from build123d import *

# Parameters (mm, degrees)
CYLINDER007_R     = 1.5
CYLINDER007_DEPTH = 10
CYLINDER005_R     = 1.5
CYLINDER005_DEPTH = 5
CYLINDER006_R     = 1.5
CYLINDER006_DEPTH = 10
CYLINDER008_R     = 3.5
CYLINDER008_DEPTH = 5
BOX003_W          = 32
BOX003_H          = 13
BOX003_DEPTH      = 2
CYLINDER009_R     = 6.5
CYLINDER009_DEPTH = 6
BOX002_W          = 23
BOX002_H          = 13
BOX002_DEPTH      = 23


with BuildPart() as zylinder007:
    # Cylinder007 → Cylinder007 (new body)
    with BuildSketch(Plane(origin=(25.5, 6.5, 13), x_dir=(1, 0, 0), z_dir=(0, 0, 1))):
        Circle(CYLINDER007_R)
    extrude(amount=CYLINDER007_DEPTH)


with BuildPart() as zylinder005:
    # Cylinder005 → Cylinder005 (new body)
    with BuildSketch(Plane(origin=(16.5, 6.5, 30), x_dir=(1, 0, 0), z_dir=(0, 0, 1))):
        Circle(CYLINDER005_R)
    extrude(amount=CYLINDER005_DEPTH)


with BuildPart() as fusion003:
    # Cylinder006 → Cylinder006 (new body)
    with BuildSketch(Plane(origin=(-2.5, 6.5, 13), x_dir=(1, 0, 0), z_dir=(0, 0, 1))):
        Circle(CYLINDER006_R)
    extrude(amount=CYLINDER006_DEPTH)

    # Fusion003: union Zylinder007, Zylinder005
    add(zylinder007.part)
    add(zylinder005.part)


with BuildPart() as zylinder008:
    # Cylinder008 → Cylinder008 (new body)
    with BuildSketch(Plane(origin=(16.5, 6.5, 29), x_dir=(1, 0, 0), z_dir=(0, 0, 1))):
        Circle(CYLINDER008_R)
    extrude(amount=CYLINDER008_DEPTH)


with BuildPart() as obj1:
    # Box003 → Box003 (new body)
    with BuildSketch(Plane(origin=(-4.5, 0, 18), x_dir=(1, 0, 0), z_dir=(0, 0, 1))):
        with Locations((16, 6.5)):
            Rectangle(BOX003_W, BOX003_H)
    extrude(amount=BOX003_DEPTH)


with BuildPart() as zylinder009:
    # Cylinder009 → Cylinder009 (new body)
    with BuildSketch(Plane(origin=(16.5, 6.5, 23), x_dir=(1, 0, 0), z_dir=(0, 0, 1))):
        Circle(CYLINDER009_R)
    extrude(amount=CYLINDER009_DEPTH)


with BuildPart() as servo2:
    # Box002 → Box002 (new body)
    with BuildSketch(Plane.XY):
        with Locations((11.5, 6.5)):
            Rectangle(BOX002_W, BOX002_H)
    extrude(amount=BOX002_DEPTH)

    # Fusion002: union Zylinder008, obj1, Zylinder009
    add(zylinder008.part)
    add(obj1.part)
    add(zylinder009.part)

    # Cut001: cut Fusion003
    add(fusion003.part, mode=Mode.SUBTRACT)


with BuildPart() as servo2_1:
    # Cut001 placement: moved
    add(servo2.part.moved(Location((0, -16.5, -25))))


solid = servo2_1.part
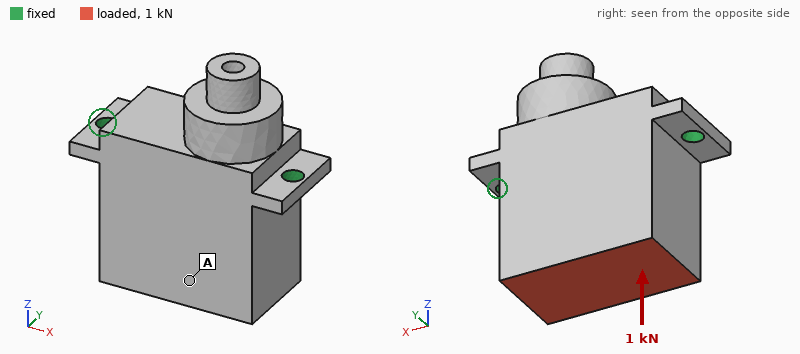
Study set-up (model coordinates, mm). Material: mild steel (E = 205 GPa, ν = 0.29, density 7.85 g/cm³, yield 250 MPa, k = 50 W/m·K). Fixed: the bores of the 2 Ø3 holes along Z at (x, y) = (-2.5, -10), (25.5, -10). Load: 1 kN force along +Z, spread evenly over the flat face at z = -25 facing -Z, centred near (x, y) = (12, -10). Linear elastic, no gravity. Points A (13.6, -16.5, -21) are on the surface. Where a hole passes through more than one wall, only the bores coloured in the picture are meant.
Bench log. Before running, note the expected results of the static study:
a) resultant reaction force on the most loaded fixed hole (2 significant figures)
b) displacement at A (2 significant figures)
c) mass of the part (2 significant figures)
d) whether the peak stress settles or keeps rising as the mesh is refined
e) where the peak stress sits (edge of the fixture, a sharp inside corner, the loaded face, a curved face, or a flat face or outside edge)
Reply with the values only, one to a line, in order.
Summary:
500 N
2.0 µm
63 g
keeps rising
edge of the fixture
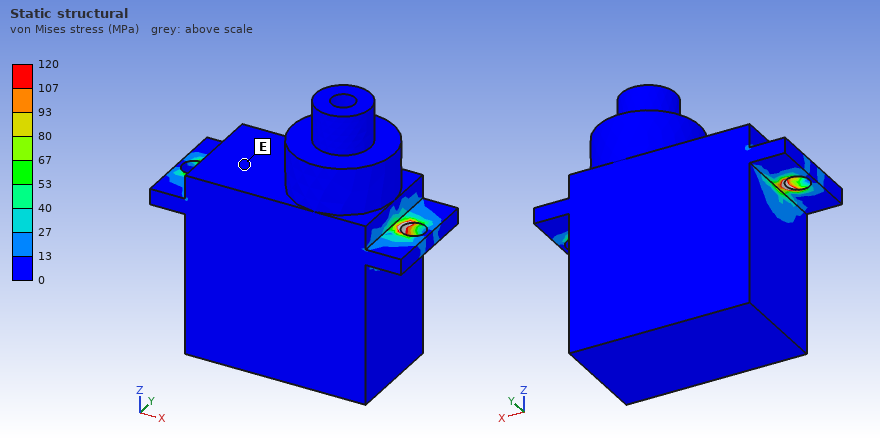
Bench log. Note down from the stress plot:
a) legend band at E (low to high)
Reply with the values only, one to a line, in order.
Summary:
0 to 13 MPa
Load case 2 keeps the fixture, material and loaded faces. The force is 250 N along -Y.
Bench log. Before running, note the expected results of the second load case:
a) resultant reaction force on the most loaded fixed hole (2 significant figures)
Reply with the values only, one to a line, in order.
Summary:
130 N
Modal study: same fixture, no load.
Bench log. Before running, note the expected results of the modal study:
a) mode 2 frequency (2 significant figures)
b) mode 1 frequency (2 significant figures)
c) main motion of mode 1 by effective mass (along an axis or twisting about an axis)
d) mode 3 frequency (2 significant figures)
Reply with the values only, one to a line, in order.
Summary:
14 kHz
3200 Hz
along Y
15 kHz
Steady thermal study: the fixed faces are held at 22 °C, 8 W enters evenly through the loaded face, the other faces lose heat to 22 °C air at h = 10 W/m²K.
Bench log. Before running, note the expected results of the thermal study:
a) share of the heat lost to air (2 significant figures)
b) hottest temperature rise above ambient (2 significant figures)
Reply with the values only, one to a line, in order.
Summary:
4.6 %
23 K
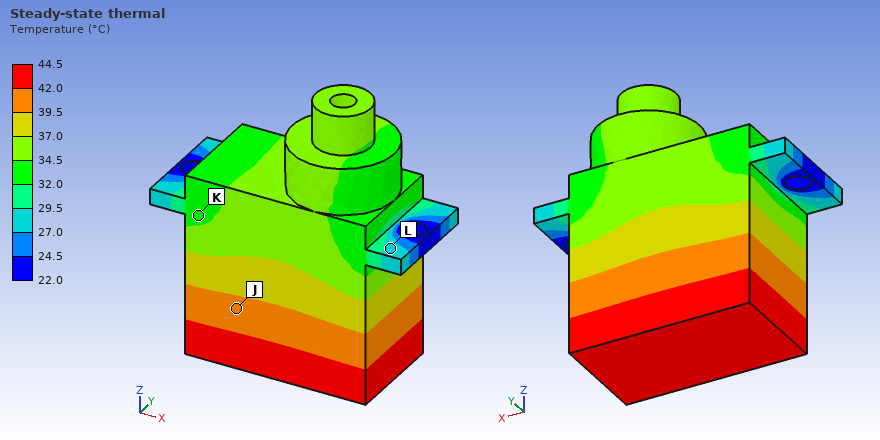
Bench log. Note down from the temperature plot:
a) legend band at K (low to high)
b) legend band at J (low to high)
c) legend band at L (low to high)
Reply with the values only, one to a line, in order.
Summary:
32.0 to 34.5 °C
39.5 to 42.0 °C
27.0 to 29.5 °C
